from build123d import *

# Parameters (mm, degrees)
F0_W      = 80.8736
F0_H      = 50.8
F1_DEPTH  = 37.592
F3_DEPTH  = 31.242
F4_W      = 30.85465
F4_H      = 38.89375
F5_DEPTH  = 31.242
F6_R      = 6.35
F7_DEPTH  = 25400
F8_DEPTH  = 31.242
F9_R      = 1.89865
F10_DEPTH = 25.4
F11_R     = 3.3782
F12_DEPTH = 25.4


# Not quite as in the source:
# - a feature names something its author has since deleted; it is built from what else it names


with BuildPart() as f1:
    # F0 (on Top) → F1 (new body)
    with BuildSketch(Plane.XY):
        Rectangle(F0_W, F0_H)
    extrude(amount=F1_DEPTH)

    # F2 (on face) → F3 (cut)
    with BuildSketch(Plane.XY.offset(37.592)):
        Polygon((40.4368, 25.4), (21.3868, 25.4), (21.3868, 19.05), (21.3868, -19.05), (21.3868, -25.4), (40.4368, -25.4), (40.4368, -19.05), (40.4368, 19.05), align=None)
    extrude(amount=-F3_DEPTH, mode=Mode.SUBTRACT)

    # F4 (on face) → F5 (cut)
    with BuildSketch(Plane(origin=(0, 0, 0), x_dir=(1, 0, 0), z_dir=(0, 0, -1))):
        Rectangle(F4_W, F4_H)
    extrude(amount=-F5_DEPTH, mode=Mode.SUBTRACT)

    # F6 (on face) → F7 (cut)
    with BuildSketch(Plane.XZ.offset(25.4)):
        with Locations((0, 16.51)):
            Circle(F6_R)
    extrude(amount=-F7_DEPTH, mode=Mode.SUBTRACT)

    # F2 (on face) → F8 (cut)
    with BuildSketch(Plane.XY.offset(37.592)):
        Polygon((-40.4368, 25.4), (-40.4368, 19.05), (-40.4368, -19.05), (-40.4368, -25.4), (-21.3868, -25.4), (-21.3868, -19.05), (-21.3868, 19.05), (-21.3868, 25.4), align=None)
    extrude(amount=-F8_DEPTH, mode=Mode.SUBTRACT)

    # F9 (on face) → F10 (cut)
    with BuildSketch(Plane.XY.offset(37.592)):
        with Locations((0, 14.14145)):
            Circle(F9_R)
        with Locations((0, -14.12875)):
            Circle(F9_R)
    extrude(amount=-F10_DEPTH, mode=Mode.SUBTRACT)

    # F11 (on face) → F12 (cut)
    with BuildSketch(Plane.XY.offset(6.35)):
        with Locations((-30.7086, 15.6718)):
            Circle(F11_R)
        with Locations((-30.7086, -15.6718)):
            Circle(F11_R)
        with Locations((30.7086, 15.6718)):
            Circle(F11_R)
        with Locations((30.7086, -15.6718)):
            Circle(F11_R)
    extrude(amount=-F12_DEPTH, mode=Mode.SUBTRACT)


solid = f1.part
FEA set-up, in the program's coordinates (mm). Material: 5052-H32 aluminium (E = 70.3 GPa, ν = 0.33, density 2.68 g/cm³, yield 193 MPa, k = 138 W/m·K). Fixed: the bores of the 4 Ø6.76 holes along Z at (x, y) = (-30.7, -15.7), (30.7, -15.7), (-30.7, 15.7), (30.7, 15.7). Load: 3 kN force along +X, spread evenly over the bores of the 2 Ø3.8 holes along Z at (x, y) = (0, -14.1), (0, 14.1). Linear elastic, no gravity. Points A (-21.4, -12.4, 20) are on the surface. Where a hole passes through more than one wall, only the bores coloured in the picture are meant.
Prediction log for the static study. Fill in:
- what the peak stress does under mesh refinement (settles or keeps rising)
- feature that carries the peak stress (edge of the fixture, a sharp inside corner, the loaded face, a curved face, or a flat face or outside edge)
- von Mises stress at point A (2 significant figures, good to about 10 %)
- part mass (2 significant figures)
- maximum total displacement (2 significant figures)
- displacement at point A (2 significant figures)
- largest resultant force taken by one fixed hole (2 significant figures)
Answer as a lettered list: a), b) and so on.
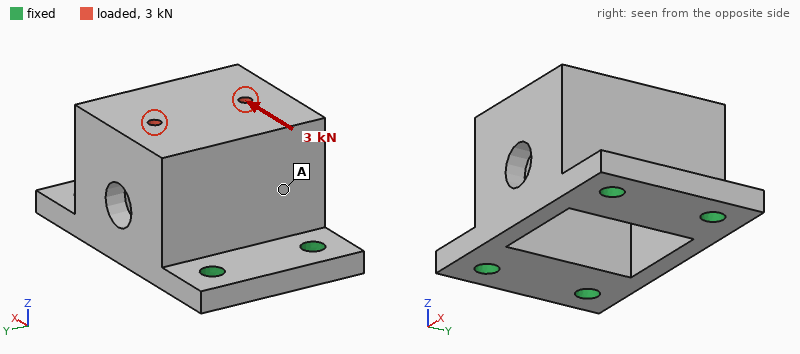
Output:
a) keeps rising
b) edge of the fixture
c) 4.0 MPa
d) 140 g
e) 23 µm
f) 12 µm
g) 1.2 kN
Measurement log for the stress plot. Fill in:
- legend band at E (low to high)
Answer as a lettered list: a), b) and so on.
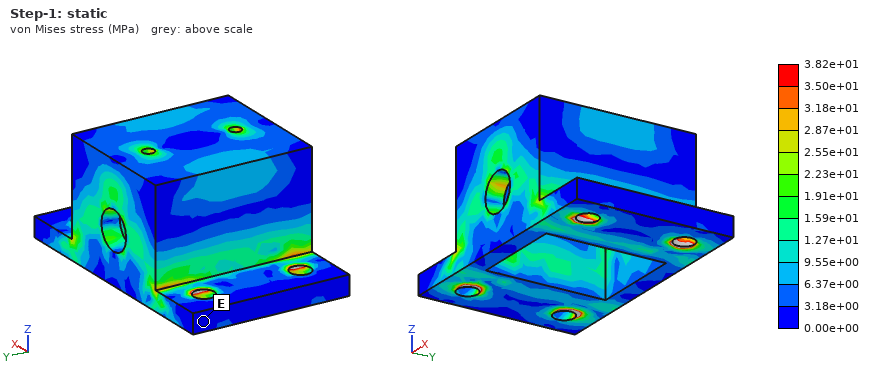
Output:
a) 0.00e+00 to 3.18e+00 MPa
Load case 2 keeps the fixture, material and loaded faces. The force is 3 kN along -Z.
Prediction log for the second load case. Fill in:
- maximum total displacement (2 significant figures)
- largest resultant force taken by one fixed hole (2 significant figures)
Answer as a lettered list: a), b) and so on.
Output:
a) 19 µm
b) 810 N
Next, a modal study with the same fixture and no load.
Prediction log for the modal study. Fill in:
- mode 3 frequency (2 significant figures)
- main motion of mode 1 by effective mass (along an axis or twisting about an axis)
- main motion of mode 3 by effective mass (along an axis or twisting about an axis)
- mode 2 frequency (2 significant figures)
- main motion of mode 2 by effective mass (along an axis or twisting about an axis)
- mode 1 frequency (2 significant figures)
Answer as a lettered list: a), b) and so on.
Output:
a) 9500 Hz
b) along Y
c) along Z
d) 7900 Hz
e) along X
f) 5600 Hz
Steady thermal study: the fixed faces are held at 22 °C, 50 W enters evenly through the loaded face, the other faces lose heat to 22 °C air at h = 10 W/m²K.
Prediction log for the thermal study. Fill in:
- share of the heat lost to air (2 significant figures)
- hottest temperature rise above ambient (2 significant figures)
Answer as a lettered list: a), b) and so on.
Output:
a) 4.4 %
b) 29 K
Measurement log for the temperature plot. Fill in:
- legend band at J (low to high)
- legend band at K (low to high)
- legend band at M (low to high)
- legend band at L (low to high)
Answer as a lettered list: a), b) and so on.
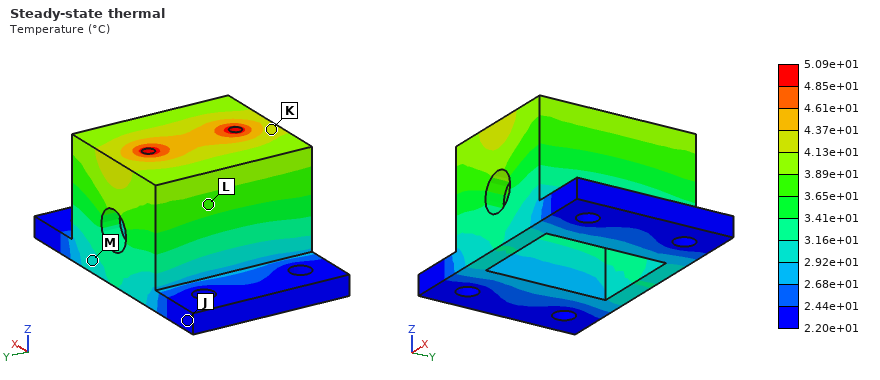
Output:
a) 2.20e+01 to 2.44e+01 °C
b) 4.13e+01 to 4.37e+01 °C
c) 2.92e+01 to 3.16e+01 °C
d) 3.65e+01 to 3.89e+01 °C
